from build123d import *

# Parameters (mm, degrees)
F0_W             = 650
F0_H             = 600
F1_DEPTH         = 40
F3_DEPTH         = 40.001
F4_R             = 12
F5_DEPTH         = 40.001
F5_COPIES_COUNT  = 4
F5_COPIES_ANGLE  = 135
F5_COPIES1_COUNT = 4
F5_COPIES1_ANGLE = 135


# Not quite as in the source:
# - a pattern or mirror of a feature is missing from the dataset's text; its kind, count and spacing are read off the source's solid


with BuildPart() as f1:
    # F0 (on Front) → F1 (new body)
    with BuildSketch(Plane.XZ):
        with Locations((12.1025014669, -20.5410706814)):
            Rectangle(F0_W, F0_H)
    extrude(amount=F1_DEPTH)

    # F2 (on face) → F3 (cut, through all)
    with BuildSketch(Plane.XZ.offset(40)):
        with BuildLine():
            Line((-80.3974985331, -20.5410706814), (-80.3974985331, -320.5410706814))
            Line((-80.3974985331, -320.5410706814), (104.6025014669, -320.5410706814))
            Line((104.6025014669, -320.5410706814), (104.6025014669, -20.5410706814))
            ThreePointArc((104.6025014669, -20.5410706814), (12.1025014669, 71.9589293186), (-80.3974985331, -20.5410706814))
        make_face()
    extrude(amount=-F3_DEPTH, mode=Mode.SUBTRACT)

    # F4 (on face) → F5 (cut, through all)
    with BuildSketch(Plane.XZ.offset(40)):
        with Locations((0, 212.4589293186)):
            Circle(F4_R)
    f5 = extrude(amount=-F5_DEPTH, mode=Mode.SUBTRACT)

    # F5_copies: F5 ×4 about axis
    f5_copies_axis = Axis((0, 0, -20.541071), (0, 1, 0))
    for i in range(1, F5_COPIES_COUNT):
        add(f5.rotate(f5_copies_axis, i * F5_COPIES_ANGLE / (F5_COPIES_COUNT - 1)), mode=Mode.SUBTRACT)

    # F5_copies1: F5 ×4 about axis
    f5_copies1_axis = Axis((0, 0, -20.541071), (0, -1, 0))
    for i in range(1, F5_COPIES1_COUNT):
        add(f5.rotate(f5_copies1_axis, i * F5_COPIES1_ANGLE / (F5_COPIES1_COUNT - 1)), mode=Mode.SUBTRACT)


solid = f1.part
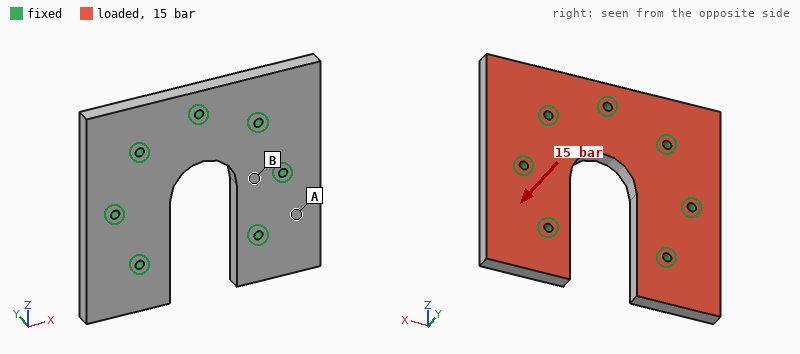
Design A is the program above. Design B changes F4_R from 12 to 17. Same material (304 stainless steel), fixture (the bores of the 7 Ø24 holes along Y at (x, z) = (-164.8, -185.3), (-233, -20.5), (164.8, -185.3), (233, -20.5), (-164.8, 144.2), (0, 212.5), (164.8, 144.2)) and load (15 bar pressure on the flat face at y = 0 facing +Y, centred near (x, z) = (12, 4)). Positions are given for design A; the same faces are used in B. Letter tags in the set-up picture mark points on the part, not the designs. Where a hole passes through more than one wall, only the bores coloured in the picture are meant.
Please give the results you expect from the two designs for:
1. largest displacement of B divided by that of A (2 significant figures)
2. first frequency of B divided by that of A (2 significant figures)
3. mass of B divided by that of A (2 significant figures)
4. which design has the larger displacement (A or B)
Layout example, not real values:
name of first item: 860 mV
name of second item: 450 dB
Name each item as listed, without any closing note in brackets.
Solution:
largest displacement of B divided by that of A: 0.85
first frequency of B divided by that of A: 1.1
mass of B divided by that of A: 0.99
which design has the larger displacement: A
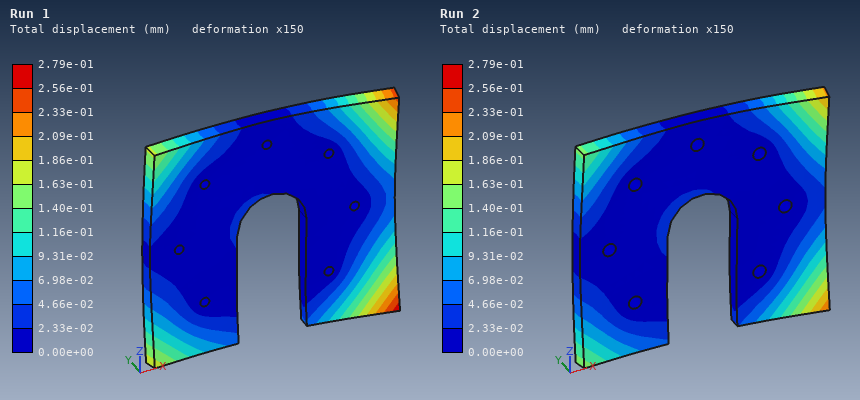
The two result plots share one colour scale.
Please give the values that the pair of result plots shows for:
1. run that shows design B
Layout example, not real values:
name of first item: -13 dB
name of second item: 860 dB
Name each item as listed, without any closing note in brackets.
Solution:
run that shows design B: Run 2
